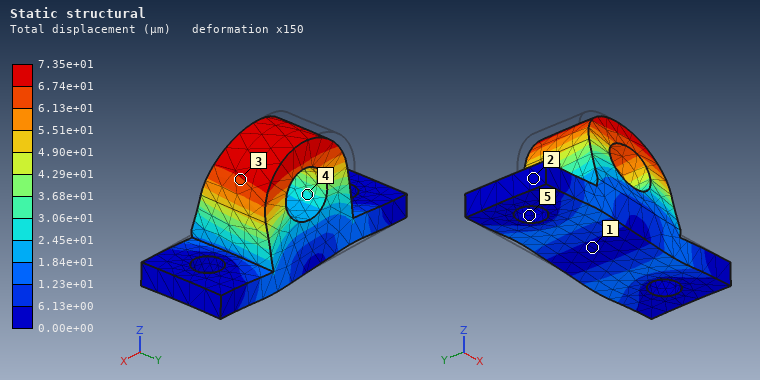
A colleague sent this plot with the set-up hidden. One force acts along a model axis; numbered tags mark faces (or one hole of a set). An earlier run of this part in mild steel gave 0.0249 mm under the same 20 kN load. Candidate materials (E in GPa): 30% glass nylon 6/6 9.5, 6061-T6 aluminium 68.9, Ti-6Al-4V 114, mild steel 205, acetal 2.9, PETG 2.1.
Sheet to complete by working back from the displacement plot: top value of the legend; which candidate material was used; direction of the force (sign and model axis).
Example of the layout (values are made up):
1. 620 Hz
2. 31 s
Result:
1. 7.35e+01 µm
2. 6061-T6 aluminium
3. +X
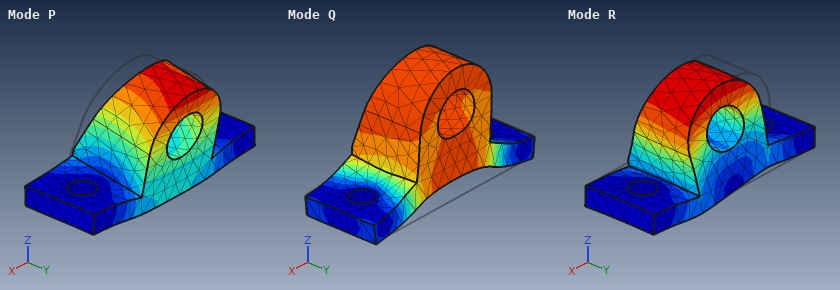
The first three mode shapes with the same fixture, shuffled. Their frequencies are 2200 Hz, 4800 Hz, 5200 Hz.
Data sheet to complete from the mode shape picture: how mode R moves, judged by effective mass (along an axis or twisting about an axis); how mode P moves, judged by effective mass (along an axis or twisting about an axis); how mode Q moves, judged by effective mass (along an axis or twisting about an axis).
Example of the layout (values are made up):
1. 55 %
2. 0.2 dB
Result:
1. along X
2. along Y
3. along Z
